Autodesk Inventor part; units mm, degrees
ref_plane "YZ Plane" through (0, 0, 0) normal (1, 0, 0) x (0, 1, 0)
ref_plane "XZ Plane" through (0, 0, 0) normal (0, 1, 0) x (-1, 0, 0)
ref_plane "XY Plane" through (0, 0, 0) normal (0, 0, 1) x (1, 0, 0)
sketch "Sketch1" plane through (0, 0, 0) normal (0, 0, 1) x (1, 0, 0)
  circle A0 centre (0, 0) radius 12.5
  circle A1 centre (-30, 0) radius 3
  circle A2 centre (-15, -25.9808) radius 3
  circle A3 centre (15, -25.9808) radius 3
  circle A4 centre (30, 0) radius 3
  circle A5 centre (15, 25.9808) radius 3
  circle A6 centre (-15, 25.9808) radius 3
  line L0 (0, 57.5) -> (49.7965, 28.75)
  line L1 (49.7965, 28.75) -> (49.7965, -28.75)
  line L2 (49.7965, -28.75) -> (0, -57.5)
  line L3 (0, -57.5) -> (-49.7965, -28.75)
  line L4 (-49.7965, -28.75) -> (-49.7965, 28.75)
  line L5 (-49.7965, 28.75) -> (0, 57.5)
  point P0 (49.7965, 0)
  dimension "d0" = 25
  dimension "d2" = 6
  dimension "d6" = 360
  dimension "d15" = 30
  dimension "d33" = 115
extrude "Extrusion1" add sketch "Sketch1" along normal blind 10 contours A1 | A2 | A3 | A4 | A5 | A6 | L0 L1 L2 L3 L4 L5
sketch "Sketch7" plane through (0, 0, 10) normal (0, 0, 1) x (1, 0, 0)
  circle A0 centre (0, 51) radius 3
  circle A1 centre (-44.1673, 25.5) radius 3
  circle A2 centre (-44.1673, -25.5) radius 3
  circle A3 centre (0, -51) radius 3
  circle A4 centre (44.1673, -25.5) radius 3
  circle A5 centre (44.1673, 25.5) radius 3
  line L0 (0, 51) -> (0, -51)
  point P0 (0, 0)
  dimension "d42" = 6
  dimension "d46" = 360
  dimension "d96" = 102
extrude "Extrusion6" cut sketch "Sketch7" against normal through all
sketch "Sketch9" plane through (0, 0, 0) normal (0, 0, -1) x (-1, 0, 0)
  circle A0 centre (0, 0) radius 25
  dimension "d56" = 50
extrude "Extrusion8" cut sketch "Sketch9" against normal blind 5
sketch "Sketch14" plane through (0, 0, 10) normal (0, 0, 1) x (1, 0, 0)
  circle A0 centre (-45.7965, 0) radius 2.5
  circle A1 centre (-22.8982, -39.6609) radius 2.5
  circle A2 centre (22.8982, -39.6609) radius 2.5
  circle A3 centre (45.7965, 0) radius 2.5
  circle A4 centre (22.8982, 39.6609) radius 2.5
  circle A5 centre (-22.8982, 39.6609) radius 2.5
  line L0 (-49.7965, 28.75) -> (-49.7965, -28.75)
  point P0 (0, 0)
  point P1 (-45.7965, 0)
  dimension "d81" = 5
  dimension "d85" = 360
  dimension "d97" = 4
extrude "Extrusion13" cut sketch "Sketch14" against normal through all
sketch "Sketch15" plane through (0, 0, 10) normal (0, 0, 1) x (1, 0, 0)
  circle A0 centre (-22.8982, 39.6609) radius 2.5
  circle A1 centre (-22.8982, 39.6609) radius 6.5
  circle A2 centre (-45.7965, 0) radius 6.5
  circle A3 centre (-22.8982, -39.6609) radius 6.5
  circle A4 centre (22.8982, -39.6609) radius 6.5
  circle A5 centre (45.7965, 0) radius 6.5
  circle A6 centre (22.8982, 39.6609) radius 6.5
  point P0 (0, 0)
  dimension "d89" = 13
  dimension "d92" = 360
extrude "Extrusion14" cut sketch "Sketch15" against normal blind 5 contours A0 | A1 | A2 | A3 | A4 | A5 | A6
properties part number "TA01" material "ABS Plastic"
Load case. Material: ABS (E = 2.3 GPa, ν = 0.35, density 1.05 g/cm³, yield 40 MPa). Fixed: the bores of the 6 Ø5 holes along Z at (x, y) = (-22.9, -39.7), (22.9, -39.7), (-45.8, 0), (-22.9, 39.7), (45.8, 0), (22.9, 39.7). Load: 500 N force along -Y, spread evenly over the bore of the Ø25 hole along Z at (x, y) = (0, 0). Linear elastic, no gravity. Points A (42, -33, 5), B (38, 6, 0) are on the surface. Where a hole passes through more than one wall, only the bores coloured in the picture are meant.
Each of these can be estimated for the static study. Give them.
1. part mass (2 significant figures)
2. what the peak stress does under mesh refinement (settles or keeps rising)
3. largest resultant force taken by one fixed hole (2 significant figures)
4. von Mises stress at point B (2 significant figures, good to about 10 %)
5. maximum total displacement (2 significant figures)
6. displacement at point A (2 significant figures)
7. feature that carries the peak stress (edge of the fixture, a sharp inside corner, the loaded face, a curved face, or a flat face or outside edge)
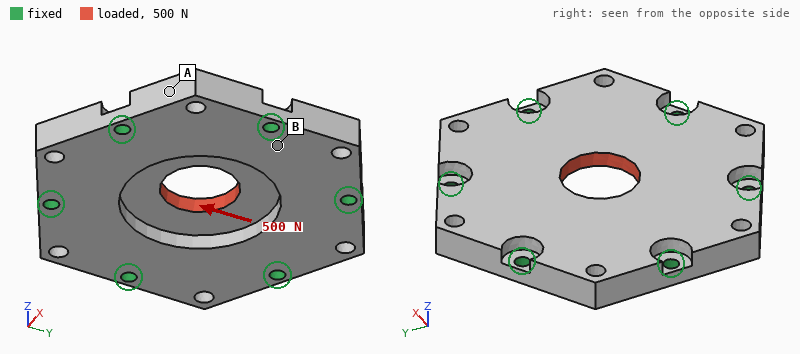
71 g
keeps rising
100 N
0.58 MPa
28 µm
7.3 µm
edge of the fixture
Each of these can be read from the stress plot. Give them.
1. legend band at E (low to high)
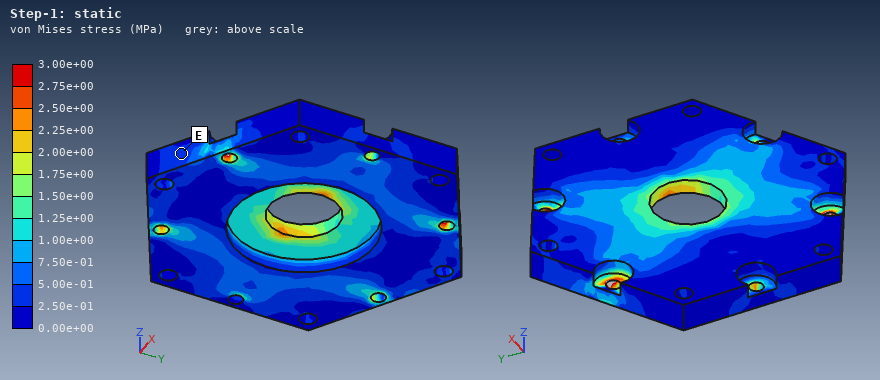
2.50e-01 to 5.00e-01 MPa
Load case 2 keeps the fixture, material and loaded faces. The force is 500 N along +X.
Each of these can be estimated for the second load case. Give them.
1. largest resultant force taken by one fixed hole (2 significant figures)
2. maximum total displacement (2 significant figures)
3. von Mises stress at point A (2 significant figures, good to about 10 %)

110 N
28 µm
0.27 MPa
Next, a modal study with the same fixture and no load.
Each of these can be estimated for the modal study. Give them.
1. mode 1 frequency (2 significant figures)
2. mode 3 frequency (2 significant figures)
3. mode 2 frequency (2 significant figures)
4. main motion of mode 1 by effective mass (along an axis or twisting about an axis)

2300 Hz
3400 Hz
3400 Hz
along Z
